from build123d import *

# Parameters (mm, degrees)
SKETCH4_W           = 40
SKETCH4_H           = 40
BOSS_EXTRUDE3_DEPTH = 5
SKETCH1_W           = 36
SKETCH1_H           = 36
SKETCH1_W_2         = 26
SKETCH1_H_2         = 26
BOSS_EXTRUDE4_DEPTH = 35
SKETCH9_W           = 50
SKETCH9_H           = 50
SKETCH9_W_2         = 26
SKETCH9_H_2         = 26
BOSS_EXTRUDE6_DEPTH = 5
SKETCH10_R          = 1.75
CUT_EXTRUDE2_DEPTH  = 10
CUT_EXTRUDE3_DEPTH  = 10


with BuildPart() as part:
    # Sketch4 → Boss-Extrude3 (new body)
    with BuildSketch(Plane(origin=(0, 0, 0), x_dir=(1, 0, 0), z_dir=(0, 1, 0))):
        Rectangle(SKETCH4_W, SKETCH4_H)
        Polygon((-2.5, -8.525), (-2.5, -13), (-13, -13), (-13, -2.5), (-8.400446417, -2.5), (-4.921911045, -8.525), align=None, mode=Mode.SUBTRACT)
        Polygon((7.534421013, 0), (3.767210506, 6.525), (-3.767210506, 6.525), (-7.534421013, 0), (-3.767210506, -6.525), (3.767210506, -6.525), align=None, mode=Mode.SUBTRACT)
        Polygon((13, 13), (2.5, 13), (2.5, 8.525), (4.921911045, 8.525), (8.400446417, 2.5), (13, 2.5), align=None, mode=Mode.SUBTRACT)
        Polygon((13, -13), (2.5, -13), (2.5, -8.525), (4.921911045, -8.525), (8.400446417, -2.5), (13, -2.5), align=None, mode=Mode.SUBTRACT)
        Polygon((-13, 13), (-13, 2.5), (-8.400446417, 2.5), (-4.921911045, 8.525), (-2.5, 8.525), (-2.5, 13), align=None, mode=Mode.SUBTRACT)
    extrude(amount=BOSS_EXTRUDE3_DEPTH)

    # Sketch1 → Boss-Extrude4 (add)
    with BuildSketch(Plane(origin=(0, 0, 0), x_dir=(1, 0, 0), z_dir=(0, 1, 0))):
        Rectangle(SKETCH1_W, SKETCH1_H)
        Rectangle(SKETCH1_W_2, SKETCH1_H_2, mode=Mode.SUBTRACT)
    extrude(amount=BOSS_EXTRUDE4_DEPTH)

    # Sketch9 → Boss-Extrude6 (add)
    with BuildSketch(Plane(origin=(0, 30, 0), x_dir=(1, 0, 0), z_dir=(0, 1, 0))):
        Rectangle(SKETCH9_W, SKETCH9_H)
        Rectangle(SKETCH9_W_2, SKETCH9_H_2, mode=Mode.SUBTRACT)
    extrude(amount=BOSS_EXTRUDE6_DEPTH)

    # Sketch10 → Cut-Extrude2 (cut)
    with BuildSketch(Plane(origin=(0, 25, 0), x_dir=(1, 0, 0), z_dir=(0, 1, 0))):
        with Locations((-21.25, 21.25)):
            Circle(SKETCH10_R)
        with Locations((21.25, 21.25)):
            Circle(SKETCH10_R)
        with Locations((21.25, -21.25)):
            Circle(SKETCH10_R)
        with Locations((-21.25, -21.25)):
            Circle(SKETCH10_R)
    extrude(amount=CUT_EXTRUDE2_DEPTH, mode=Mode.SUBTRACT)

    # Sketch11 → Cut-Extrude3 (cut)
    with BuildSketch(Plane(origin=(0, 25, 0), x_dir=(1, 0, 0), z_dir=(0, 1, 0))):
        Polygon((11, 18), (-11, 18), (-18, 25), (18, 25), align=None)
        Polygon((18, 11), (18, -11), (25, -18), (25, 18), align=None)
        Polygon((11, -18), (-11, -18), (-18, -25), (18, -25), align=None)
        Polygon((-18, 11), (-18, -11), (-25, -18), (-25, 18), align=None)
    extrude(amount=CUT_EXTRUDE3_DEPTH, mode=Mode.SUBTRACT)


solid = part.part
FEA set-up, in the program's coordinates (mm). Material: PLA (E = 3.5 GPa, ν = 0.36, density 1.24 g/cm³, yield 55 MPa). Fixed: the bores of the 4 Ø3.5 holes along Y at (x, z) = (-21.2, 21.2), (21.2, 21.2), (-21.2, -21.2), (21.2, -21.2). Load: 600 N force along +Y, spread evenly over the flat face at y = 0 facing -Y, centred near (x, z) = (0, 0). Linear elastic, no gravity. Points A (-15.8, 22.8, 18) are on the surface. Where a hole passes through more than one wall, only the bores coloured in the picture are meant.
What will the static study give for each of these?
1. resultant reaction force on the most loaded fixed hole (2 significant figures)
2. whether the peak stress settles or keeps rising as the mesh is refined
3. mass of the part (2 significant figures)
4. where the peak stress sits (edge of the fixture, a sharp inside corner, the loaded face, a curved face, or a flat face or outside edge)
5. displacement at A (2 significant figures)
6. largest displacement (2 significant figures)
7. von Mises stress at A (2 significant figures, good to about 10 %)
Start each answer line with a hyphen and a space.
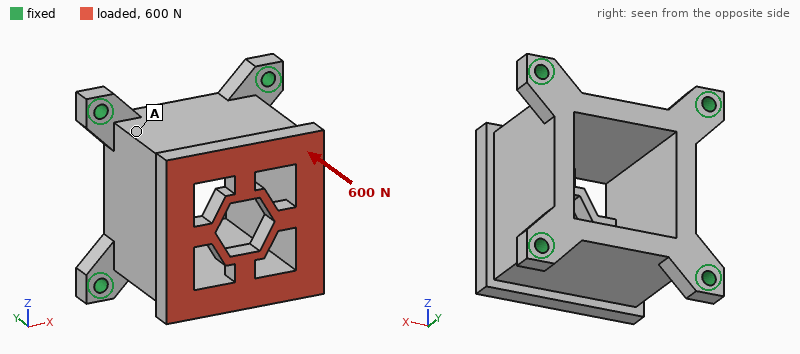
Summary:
- 170 N
- keeps rising
- 32 g
- edge of the fixture
- 44 µm
- 68 µm
- 3.1 MPa
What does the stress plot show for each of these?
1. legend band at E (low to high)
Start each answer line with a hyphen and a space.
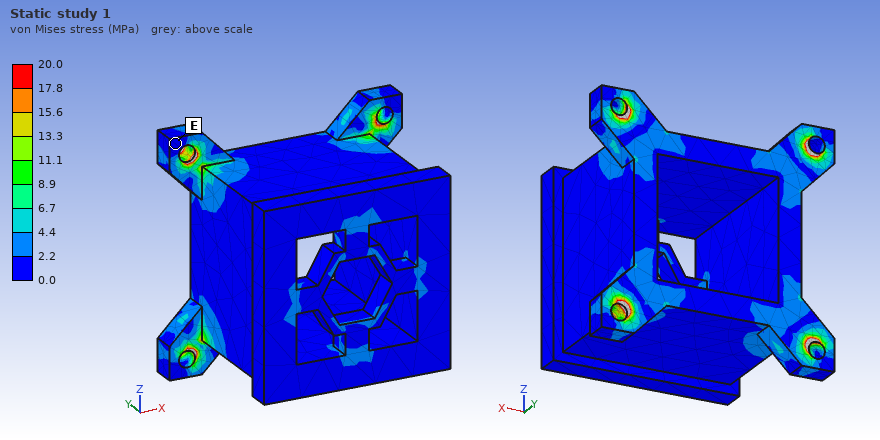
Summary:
- 0.0 to 2.2 MPa
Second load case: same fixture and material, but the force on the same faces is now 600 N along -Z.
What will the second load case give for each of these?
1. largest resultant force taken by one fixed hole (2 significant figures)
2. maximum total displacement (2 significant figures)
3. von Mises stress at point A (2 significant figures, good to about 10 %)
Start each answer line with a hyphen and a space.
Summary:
- 320 N
- 0.24 mm
- 5.6 MPa
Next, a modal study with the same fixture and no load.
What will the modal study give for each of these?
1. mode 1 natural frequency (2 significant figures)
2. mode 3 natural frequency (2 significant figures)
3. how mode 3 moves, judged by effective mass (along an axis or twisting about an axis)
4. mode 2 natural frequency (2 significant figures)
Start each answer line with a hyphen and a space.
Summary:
- 2400 Hz
- 3300 Hz
- along Y
- 2400 Hz
